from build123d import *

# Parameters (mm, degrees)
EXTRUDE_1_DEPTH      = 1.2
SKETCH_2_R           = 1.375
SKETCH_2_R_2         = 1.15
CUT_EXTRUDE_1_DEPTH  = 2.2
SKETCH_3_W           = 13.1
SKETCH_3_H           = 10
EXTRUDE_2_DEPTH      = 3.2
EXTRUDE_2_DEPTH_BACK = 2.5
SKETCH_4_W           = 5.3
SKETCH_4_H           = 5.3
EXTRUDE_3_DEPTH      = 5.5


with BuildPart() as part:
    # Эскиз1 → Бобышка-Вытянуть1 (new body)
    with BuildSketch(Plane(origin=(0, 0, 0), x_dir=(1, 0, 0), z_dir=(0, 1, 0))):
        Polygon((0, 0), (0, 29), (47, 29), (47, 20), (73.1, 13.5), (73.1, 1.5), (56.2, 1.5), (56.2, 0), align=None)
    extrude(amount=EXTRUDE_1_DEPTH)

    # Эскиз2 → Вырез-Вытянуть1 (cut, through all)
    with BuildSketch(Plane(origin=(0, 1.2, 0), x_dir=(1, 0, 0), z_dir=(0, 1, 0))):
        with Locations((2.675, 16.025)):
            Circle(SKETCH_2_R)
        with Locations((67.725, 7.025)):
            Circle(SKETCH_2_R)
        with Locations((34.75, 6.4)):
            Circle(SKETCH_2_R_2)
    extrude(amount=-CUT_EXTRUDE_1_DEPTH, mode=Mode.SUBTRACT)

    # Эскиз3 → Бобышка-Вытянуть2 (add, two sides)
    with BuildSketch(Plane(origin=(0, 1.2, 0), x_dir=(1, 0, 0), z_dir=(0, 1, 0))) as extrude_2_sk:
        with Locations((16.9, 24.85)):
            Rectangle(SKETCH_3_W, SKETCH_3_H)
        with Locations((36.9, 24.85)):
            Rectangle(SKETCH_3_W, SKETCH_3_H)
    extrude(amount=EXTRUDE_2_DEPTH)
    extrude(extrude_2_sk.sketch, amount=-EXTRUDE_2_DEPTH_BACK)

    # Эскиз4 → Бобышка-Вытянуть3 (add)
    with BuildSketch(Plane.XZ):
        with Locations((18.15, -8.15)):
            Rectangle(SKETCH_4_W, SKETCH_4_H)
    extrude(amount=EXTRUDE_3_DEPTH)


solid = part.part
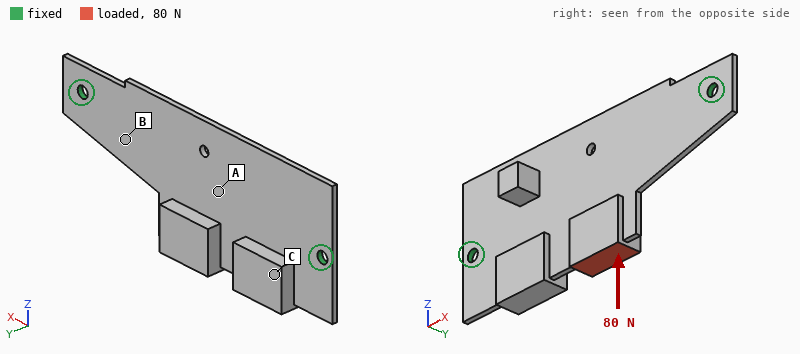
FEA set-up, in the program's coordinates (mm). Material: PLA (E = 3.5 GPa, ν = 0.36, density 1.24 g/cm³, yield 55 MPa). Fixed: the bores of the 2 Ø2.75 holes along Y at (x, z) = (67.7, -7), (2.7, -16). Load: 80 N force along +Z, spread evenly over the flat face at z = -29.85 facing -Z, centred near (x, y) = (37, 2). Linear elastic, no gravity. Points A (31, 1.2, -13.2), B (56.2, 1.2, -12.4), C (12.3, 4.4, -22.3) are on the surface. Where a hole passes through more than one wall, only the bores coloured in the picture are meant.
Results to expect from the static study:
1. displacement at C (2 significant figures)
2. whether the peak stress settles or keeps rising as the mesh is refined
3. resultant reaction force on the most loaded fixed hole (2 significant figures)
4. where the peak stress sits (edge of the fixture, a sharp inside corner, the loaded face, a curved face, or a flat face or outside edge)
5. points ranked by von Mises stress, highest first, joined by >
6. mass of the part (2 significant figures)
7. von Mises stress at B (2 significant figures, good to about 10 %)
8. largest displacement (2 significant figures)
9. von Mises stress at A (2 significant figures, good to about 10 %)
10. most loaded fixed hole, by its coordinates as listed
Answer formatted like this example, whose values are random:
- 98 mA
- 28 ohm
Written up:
- 0.28 mm
- keeps rising
- 46 N
- edge of the fixture
- B > A > C
- 4.3 g
- 9.1 MPa
- 0.94 mm
- 3.9 MPa
- (67.7, -7)
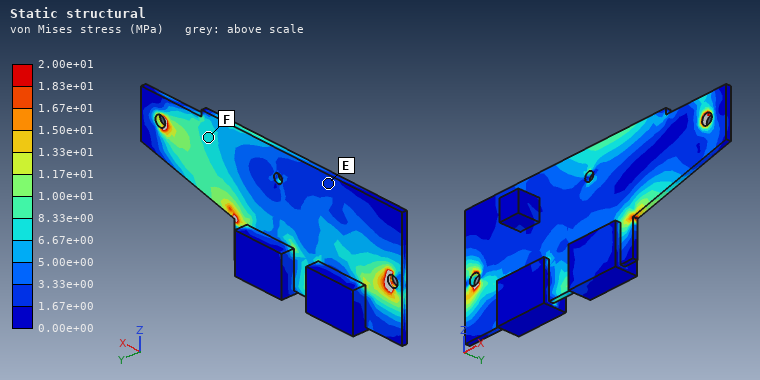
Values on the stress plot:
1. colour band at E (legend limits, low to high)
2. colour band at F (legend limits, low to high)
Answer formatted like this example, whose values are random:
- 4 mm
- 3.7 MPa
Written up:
- 1.67e+00 to 3.33e+00 MPa
- 6.67e+00 to 8.33e+00 MPa
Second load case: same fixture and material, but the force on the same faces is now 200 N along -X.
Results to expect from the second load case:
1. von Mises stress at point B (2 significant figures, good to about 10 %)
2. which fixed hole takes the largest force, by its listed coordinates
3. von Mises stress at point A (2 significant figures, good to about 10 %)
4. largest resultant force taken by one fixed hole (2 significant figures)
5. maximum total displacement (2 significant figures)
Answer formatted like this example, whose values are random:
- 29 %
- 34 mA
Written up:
- 9.1 MPa
- (2.7, -16)
- 6.7 MPa
- 140 N
- 0.95 mm
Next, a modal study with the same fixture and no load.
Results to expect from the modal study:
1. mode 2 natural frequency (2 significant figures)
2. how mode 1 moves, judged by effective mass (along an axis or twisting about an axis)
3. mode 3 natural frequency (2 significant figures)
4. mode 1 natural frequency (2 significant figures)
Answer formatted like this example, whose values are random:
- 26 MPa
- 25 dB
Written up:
- 520 Hz
- along Y
- 1000 Hz
- 290 Hz
